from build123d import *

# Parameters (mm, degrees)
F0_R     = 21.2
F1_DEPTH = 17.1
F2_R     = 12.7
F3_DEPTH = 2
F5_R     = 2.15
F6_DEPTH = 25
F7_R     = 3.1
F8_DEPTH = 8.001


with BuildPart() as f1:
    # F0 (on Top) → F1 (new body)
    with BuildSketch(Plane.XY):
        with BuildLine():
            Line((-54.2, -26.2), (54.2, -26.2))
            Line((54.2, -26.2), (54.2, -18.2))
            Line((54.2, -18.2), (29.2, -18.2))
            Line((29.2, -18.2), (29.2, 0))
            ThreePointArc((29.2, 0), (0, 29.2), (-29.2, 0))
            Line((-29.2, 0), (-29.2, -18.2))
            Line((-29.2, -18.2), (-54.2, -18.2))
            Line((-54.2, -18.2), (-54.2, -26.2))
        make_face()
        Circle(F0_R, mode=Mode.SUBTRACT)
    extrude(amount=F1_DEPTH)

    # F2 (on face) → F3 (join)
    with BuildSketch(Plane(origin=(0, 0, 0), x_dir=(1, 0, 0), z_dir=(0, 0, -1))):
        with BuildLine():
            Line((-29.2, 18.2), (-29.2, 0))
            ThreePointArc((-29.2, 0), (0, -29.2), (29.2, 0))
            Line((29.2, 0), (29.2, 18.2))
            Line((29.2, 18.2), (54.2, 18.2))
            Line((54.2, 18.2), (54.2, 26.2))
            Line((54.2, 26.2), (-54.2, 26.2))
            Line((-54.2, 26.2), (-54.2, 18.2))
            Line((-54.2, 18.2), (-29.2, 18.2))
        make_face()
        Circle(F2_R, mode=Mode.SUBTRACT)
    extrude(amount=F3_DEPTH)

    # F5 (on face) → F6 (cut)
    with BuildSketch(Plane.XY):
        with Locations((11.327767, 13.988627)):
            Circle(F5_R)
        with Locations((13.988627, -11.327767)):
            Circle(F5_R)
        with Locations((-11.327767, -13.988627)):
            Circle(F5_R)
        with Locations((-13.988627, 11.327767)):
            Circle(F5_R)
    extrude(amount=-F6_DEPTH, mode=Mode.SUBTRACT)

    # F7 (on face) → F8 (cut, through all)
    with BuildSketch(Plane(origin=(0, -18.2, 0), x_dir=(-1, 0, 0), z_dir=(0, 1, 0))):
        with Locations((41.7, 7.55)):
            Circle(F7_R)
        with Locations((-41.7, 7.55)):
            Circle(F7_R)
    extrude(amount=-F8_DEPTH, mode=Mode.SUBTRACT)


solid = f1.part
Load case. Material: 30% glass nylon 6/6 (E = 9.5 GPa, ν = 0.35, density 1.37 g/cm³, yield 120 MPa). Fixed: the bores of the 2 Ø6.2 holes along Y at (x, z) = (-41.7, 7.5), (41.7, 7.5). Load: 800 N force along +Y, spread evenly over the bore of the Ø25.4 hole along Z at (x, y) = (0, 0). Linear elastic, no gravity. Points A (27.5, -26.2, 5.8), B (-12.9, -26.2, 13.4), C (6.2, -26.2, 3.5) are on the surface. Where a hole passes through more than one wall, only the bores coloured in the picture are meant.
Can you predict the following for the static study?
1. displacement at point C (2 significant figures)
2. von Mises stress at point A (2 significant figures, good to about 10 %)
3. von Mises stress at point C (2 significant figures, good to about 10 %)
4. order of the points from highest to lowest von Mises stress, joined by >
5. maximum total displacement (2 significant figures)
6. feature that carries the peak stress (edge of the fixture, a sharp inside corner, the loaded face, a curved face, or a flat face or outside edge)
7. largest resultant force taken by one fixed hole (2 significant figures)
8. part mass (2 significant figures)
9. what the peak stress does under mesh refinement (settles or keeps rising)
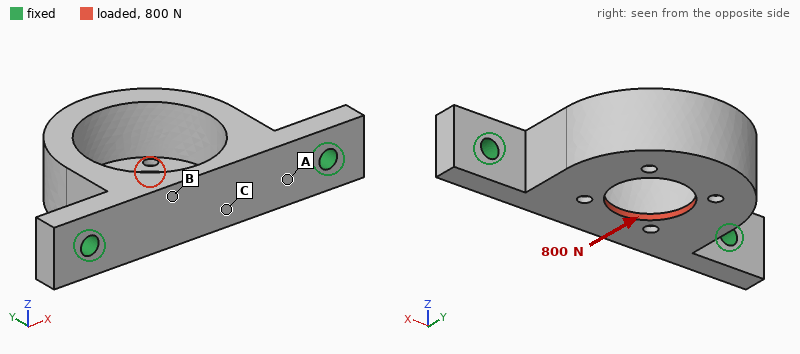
0.086 mm
9.5 MPa
5.3 MPa
A > C > B
0.31 mm
edge of the fixture
420 N
50 g
keeps rising
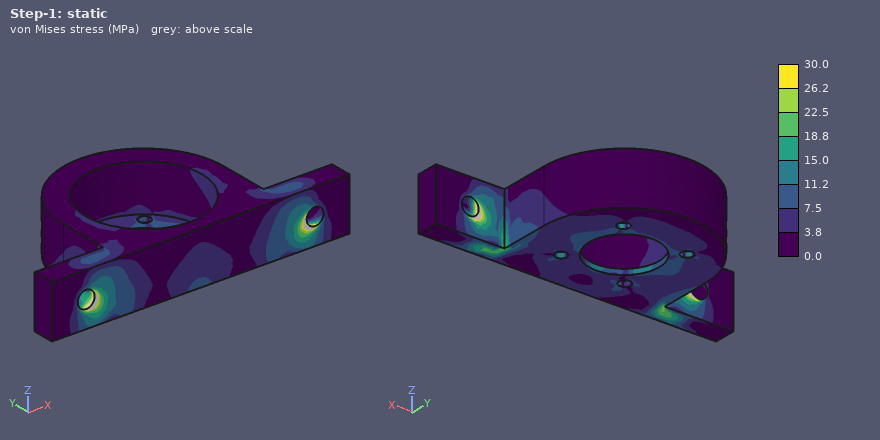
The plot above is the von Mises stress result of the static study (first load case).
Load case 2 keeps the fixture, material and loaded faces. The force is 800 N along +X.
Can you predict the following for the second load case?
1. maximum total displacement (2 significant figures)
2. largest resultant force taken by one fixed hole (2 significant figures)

89 µm
480 N
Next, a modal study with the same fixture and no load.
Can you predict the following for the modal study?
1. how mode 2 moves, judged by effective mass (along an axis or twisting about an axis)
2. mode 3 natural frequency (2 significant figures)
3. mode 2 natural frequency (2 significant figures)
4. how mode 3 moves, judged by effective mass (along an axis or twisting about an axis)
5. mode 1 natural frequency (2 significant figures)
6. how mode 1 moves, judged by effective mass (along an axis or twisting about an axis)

along X
3300 Hz
2700 Hz
along Y
1000 Hz
along Z
